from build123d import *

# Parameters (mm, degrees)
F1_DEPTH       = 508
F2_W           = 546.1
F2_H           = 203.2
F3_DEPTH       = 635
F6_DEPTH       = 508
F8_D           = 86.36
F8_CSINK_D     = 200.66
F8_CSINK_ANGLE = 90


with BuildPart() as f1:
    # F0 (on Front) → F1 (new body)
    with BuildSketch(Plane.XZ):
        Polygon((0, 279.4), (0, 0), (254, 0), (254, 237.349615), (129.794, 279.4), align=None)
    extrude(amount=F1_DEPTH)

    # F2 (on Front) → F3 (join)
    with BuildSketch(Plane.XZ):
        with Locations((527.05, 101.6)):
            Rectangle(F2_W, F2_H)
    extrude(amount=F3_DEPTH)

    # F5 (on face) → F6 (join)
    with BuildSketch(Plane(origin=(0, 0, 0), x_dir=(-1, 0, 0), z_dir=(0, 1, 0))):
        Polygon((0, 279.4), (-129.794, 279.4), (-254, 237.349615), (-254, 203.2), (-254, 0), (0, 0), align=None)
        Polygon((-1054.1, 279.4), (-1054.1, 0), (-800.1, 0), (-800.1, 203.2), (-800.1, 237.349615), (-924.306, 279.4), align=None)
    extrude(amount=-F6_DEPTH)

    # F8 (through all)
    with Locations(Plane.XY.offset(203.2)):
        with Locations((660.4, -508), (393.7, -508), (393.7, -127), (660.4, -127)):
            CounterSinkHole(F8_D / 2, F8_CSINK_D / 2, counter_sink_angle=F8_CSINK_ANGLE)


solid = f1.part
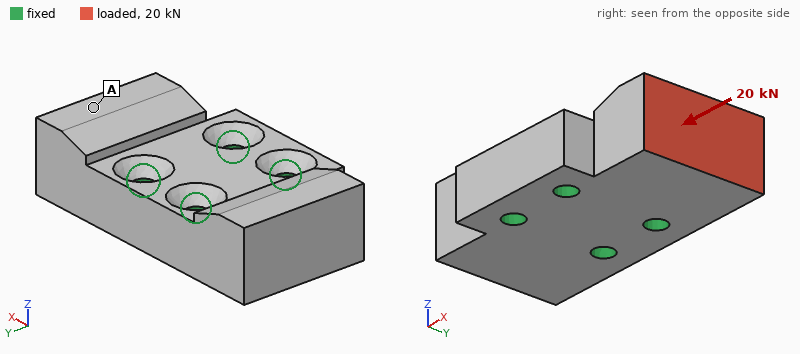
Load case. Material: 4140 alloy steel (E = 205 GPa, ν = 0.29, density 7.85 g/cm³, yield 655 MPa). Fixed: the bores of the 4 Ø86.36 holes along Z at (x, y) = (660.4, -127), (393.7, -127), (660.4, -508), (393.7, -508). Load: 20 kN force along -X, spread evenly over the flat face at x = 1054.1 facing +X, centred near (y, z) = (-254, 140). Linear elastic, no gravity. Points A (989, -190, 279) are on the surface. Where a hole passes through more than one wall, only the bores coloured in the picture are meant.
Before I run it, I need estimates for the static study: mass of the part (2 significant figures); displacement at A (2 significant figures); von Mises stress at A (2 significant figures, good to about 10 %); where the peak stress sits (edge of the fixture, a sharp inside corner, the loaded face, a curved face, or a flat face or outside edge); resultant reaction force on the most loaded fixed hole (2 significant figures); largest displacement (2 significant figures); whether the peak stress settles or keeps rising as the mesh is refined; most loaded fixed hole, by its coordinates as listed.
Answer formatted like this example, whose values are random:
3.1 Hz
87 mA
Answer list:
1000 kg
1.3 µm
0.13 MPa
edge of the fixture
10 kN
1.5 µm
keeps rising
(660.4, -127)
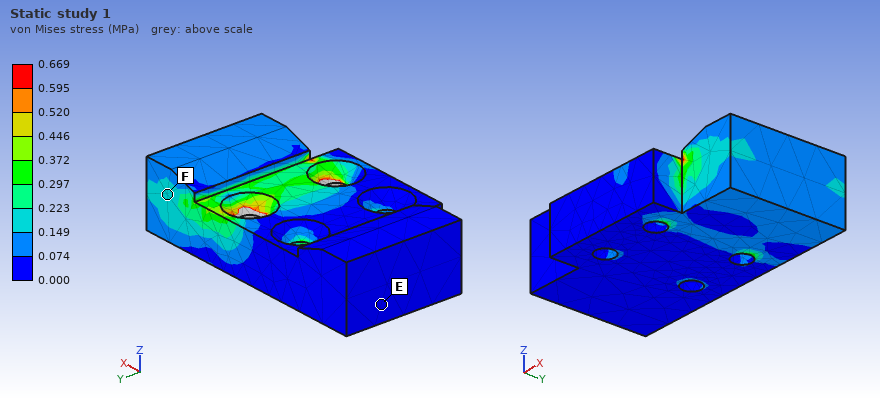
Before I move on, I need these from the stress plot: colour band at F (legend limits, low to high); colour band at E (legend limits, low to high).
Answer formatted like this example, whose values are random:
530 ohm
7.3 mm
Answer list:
0.149 to 0.223 MPa
0.000 to 0.074 MPa
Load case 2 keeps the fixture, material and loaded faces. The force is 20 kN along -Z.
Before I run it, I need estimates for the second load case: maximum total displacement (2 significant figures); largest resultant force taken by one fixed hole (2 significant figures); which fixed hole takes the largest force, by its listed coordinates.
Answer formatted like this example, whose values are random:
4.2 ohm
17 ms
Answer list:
9.2 µm
18 kN
(660.4, -127)
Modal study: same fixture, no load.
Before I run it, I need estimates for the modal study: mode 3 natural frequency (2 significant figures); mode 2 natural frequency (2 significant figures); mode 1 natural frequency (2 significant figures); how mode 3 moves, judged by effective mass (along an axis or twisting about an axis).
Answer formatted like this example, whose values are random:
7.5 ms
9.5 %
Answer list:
1300 Hz
680 Hz
660 Hz
twisting about Z
